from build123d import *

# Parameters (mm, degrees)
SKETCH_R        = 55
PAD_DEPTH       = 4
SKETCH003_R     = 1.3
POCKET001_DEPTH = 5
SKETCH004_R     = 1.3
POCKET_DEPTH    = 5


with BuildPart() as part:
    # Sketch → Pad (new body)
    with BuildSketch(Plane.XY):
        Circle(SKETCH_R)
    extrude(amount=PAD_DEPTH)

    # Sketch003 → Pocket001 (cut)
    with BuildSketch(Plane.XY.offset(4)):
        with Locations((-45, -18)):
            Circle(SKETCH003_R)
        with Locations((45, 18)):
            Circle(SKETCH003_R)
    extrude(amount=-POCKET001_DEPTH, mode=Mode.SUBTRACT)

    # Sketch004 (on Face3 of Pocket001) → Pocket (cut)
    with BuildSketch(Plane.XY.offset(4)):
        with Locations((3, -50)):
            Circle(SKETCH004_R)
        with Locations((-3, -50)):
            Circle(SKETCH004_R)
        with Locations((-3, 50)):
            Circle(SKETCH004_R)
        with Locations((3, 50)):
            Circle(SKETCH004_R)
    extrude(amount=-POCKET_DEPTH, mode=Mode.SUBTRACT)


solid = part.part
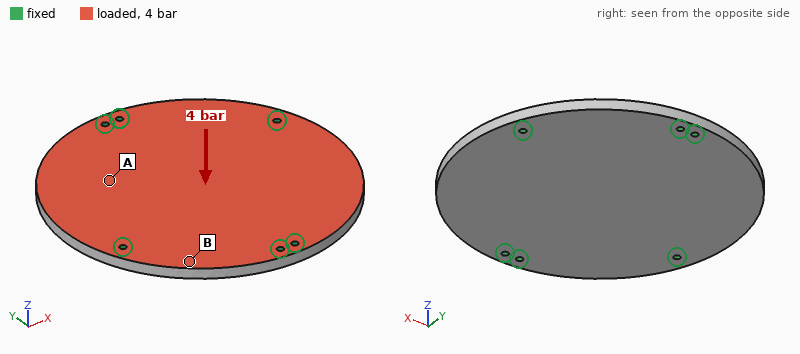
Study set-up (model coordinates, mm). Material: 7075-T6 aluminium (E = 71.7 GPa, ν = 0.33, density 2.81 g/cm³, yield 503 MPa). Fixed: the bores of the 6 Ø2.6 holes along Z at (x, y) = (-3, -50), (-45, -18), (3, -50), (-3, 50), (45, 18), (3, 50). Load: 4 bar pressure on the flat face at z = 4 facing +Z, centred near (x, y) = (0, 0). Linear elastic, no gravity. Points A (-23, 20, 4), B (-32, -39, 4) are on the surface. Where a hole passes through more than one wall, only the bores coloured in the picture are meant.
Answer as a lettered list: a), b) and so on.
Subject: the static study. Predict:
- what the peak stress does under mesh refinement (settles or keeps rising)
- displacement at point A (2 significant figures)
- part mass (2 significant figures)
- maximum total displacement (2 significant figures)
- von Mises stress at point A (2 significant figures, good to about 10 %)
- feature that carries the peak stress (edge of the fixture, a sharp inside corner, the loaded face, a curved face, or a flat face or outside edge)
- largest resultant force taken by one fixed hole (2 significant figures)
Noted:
a) keeps rising
b) 0.19 mm
c) 110 g
d) 0.25 mm
e) 52 MPa
f) edge of the fixture
g) 940 N
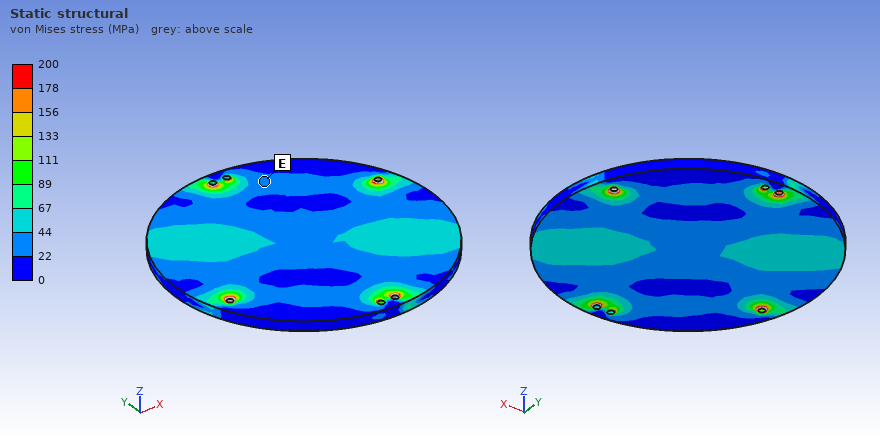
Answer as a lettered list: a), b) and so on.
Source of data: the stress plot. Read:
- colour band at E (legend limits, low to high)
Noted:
a) 22 to 44 MPa
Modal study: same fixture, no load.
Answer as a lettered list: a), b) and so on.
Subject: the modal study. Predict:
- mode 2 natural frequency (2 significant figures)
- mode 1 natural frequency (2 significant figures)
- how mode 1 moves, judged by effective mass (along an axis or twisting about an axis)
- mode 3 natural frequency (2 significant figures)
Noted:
a) 2400 Hz
b) 2300 Hz
c) along Z
d) 3200 Hz
